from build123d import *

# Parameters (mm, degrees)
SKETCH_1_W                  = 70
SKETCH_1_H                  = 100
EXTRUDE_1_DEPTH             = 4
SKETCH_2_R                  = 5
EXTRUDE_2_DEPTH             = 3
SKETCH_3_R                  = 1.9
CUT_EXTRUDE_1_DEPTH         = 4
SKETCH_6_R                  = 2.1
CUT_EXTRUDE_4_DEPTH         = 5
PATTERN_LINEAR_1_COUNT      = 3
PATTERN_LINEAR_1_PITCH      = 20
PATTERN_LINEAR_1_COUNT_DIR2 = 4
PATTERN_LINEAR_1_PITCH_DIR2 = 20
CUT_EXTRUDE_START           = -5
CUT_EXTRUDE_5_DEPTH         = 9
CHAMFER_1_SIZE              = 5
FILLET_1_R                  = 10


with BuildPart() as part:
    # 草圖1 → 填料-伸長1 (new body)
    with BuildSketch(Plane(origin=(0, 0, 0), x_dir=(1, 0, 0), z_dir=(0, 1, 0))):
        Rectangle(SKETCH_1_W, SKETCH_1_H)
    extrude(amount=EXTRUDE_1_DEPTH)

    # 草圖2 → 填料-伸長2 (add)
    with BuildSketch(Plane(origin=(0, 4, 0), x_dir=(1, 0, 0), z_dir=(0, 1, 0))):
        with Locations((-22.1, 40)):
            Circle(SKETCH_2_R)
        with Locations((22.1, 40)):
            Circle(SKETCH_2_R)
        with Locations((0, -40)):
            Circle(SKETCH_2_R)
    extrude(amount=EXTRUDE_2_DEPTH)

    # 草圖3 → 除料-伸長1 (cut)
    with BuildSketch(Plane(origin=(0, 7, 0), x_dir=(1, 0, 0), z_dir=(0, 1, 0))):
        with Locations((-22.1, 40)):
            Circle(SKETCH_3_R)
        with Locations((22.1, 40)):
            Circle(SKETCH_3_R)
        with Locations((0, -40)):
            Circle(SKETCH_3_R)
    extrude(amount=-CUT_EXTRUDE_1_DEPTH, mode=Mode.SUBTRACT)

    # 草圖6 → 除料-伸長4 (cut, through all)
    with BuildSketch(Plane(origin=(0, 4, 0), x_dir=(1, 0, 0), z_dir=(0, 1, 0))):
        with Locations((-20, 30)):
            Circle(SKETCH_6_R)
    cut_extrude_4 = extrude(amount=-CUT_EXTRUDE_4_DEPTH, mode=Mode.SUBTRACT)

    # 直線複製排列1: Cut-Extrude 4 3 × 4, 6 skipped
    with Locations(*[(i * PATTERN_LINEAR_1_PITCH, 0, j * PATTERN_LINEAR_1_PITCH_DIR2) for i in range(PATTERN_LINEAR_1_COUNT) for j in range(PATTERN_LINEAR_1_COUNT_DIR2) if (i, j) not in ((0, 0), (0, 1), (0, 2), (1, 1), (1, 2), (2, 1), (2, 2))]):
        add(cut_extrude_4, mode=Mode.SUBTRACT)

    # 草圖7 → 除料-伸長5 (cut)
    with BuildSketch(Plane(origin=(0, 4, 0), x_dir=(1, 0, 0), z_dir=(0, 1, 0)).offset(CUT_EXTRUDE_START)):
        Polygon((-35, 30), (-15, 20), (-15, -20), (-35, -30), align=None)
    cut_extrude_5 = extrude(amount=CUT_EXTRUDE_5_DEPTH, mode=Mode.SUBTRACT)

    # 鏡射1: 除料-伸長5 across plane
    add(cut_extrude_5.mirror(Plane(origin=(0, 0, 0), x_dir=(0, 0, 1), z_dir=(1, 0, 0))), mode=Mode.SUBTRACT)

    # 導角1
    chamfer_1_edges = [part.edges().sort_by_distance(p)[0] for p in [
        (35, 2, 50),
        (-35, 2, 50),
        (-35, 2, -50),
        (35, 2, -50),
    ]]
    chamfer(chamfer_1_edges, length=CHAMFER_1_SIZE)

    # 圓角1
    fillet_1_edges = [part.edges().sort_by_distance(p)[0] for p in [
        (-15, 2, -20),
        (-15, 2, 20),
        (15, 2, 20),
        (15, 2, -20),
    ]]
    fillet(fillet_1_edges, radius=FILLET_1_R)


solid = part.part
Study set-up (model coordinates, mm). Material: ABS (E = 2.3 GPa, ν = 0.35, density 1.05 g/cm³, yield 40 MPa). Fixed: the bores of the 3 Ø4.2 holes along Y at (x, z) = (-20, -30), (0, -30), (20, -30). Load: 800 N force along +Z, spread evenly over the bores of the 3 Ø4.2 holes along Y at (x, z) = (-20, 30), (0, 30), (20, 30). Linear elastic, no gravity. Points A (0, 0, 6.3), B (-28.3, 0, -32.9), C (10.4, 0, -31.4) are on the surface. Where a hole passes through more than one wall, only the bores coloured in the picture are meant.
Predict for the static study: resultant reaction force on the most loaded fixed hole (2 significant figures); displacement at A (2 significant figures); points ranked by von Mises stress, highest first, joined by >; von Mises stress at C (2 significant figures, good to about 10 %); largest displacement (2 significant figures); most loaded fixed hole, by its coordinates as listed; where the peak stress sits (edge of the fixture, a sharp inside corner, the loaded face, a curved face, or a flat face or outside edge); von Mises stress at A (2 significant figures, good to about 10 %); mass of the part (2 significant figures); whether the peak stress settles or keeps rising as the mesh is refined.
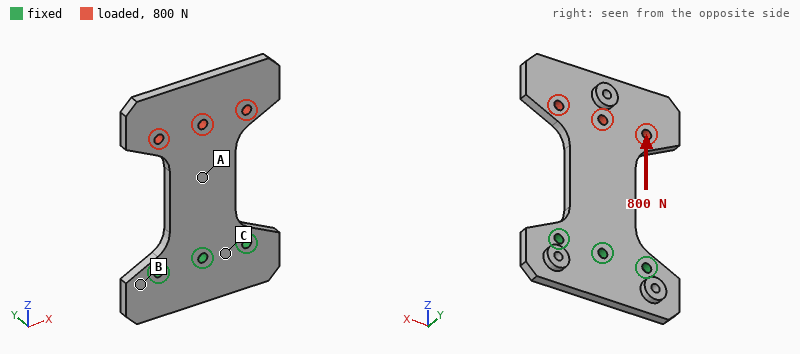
430 N
0.10 mm
A > C > B
2.3 MPa
0.20 mm
(0, -30)
edge of the fixture
6.2 MPa
21 g
keeps rising
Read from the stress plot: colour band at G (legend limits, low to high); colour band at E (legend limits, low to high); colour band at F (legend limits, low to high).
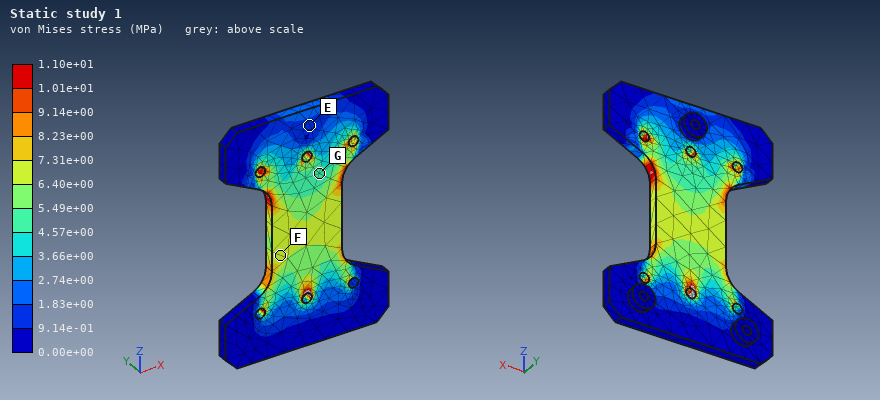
4.57e+00 to 5.49e+00 MPa
9.14e-01 to 1.83e+00 MPa
6.40e+00 to 7.31e+00 MPa
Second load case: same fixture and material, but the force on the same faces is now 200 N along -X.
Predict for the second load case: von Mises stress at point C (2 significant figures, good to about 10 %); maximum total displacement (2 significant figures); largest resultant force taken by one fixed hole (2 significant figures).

2.8 MPa
1.1 mm
320 N
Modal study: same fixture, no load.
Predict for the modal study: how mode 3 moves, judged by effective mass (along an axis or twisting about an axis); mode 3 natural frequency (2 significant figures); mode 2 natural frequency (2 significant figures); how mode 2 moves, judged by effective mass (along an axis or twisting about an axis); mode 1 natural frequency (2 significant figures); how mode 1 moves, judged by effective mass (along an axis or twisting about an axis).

along X
760 Hz
300 Hz
twisting about Z
110 Hz
along Y
